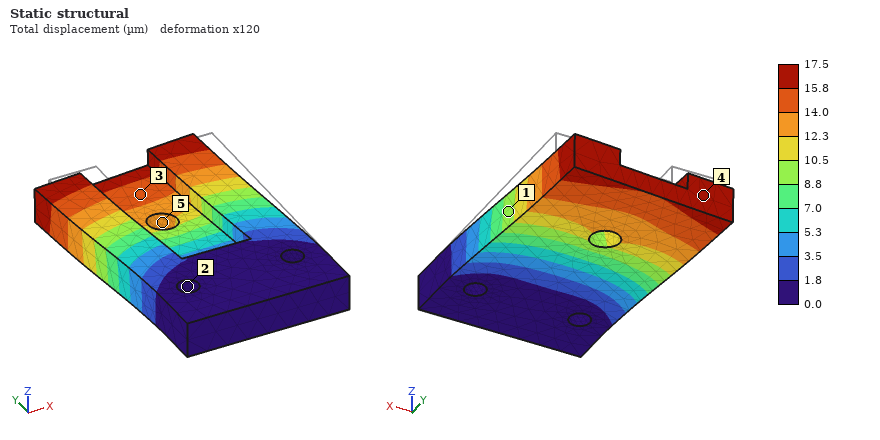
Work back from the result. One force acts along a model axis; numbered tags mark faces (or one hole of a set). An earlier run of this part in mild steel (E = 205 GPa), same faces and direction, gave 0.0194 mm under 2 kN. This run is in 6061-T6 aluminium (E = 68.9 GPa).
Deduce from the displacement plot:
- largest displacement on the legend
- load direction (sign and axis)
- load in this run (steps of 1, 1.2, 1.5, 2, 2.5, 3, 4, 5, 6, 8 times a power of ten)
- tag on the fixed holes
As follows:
17.5 µm
-X
600 N
2
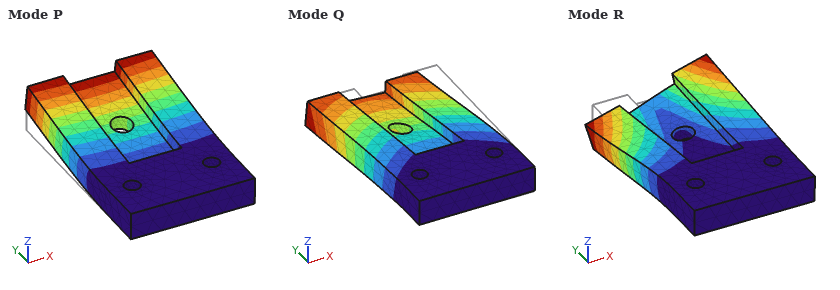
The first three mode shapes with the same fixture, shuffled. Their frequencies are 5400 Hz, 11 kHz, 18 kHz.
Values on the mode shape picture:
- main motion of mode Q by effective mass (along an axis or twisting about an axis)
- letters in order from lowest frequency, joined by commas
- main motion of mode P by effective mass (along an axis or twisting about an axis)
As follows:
along X
P, R, Q
along Z
